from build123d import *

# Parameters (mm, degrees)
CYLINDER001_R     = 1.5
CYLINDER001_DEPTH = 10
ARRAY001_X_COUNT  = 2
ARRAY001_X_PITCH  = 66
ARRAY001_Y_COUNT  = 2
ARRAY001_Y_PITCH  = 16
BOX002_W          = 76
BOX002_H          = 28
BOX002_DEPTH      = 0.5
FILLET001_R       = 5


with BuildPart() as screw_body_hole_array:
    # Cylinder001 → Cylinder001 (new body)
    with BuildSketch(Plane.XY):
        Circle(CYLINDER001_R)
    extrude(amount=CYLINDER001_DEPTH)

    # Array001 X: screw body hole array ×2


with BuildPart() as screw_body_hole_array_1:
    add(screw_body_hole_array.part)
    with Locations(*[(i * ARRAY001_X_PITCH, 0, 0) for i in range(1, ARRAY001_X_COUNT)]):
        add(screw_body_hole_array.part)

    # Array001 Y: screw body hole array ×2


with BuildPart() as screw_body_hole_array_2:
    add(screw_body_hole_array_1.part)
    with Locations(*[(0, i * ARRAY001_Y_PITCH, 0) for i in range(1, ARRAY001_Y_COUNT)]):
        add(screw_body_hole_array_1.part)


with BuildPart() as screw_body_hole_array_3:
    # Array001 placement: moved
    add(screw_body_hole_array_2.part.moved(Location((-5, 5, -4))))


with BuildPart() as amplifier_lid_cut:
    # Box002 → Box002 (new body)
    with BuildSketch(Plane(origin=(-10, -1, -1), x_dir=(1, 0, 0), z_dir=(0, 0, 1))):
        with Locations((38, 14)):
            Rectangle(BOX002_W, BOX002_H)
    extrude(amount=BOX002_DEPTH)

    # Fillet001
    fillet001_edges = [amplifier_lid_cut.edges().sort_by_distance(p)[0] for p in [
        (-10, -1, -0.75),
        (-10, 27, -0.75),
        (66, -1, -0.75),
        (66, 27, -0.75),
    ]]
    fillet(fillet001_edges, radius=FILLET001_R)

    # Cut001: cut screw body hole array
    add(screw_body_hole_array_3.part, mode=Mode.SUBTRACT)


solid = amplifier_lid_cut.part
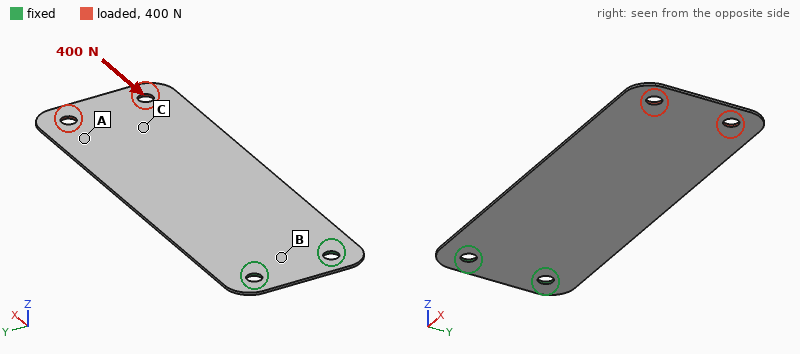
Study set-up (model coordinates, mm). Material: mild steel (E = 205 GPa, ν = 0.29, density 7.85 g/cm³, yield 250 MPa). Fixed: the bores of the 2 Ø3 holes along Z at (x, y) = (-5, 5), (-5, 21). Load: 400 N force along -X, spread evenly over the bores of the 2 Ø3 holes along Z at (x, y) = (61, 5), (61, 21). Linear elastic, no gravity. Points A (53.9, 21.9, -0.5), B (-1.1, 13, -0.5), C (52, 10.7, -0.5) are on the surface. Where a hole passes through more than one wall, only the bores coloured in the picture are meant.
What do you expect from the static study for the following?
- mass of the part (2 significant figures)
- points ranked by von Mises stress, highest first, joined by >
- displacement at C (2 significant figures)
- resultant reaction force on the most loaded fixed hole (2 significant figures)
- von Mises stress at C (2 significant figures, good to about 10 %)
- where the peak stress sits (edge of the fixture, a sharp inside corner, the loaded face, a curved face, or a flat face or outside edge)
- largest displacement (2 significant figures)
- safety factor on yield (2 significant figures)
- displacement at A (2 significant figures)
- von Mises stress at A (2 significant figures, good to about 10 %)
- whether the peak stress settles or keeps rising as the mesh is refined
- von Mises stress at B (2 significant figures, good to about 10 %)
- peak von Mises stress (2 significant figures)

8.2 g
A > C > B
8.3 µm
200 N
26 MPa
the loaded face
11 µm
2.5
8.7 µm
33 MPa
settles
15 MPa
100 MPa
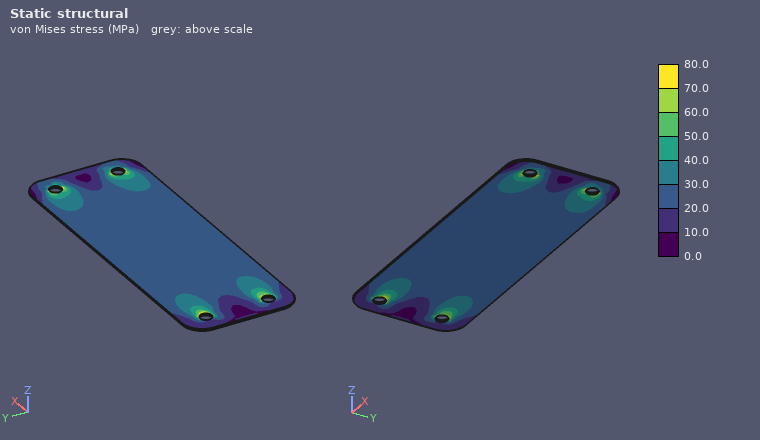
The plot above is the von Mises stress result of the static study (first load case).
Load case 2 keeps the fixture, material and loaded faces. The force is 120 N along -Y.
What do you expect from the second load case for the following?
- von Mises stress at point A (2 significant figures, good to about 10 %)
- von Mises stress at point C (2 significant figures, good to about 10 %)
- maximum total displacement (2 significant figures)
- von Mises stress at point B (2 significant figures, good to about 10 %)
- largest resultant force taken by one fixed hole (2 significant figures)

16 MPa
22 MPa
87 µm
25 MPa
450 N
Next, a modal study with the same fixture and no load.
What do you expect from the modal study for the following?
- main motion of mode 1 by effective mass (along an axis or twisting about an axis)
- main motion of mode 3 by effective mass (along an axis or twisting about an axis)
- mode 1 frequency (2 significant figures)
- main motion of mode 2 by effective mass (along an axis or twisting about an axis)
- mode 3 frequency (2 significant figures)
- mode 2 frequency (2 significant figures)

along Z
along Z
86 Hz
twisting about X
540 Hz
460 Hz
